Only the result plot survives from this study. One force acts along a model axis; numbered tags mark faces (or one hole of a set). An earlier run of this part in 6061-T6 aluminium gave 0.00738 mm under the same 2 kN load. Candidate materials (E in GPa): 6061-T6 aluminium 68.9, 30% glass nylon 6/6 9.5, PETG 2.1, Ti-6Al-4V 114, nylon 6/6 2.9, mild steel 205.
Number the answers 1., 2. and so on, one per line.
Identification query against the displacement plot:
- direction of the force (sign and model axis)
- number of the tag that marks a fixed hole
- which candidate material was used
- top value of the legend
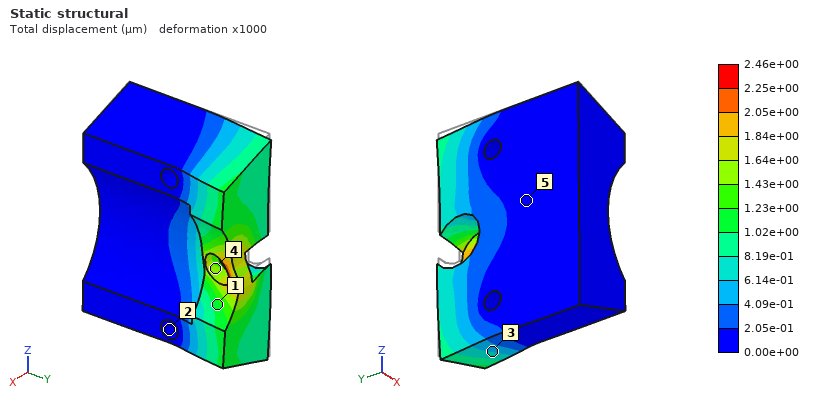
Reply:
1. -Z
2. 2
3. mild steel
4. 2.46e+00 µm
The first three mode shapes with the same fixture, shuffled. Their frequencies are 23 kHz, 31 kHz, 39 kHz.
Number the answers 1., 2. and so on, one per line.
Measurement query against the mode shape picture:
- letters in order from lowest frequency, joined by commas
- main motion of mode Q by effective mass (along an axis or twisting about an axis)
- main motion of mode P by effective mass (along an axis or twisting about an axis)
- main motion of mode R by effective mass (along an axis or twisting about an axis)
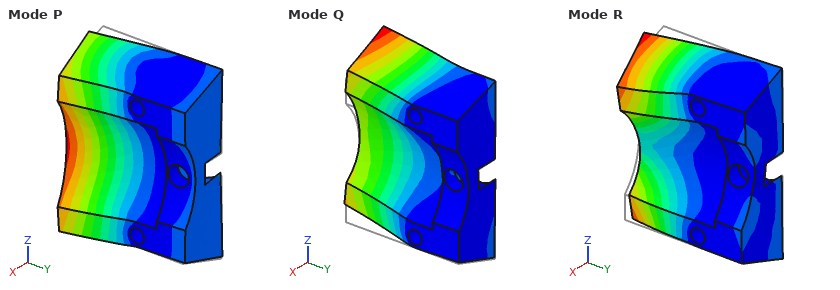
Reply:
1. P, R, Q
2. along Z
3. along X
4. twisting about Y
